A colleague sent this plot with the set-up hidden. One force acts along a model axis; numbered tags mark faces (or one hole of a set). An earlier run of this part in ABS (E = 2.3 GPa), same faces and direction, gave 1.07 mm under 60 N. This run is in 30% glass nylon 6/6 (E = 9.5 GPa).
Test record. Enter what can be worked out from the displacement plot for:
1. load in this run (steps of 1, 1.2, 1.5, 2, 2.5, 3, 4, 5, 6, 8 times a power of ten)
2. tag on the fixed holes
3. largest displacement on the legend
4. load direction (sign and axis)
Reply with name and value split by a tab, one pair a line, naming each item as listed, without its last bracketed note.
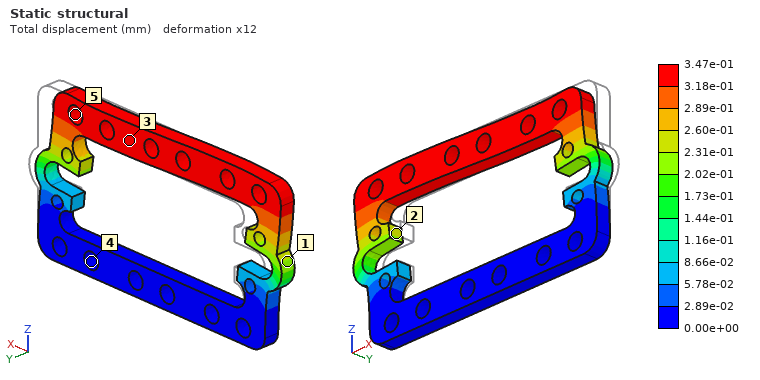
load in this run	80 N
tag on the fixed holes	4
largest displacement on the legend	3.47e-01 mm
load direction	-X
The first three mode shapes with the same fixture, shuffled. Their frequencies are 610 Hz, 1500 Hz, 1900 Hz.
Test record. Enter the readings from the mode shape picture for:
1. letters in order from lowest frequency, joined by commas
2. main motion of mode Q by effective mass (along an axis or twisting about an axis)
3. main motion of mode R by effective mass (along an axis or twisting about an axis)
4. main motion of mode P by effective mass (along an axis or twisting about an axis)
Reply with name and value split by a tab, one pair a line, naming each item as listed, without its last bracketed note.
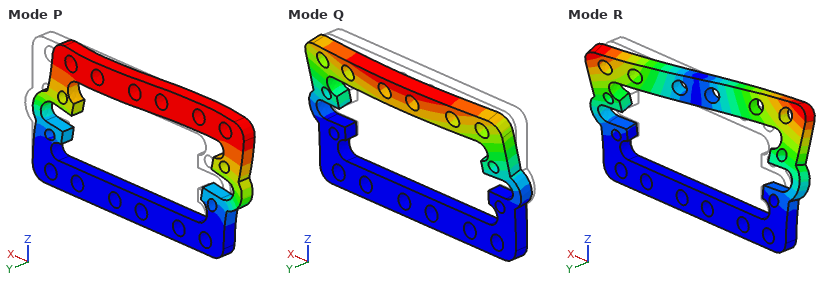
letters in order from lowest frequency, joined by commas	Q, R, P
main motion of mode Q by effective mass	along Y
main motion of mode R by effective mass	twisting about Z
main motion of mode P by effective mass	along X
